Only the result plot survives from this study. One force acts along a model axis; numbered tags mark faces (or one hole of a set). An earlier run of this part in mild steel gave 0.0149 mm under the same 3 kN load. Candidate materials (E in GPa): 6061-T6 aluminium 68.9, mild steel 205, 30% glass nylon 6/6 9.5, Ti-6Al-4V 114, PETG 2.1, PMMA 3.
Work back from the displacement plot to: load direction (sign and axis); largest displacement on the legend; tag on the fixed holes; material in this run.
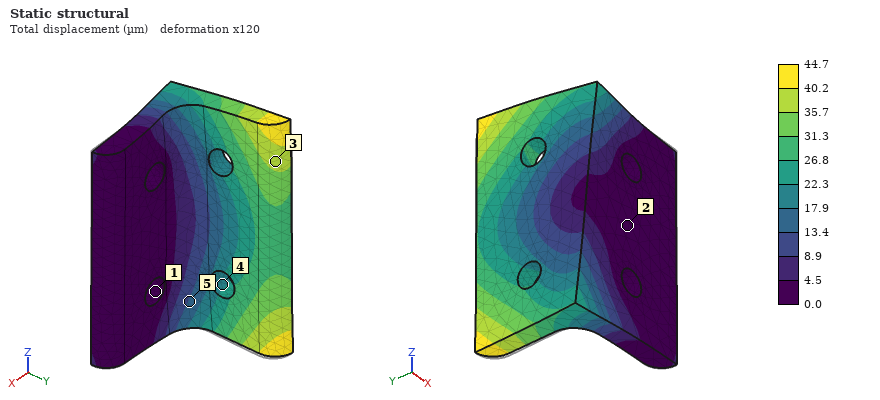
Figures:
+Z
44.7 µm
1
6061-T6 aluminium
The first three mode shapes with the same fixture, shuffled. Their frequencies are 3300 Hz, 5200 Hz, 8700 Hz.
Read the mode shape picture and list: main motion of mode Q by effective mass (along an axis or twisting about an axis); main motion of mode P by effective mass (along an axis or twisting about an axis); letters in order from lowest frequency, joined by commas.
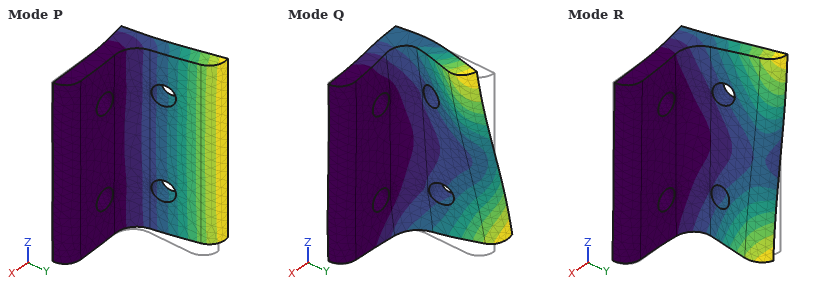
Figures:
along Z
along X
P, R, Q
